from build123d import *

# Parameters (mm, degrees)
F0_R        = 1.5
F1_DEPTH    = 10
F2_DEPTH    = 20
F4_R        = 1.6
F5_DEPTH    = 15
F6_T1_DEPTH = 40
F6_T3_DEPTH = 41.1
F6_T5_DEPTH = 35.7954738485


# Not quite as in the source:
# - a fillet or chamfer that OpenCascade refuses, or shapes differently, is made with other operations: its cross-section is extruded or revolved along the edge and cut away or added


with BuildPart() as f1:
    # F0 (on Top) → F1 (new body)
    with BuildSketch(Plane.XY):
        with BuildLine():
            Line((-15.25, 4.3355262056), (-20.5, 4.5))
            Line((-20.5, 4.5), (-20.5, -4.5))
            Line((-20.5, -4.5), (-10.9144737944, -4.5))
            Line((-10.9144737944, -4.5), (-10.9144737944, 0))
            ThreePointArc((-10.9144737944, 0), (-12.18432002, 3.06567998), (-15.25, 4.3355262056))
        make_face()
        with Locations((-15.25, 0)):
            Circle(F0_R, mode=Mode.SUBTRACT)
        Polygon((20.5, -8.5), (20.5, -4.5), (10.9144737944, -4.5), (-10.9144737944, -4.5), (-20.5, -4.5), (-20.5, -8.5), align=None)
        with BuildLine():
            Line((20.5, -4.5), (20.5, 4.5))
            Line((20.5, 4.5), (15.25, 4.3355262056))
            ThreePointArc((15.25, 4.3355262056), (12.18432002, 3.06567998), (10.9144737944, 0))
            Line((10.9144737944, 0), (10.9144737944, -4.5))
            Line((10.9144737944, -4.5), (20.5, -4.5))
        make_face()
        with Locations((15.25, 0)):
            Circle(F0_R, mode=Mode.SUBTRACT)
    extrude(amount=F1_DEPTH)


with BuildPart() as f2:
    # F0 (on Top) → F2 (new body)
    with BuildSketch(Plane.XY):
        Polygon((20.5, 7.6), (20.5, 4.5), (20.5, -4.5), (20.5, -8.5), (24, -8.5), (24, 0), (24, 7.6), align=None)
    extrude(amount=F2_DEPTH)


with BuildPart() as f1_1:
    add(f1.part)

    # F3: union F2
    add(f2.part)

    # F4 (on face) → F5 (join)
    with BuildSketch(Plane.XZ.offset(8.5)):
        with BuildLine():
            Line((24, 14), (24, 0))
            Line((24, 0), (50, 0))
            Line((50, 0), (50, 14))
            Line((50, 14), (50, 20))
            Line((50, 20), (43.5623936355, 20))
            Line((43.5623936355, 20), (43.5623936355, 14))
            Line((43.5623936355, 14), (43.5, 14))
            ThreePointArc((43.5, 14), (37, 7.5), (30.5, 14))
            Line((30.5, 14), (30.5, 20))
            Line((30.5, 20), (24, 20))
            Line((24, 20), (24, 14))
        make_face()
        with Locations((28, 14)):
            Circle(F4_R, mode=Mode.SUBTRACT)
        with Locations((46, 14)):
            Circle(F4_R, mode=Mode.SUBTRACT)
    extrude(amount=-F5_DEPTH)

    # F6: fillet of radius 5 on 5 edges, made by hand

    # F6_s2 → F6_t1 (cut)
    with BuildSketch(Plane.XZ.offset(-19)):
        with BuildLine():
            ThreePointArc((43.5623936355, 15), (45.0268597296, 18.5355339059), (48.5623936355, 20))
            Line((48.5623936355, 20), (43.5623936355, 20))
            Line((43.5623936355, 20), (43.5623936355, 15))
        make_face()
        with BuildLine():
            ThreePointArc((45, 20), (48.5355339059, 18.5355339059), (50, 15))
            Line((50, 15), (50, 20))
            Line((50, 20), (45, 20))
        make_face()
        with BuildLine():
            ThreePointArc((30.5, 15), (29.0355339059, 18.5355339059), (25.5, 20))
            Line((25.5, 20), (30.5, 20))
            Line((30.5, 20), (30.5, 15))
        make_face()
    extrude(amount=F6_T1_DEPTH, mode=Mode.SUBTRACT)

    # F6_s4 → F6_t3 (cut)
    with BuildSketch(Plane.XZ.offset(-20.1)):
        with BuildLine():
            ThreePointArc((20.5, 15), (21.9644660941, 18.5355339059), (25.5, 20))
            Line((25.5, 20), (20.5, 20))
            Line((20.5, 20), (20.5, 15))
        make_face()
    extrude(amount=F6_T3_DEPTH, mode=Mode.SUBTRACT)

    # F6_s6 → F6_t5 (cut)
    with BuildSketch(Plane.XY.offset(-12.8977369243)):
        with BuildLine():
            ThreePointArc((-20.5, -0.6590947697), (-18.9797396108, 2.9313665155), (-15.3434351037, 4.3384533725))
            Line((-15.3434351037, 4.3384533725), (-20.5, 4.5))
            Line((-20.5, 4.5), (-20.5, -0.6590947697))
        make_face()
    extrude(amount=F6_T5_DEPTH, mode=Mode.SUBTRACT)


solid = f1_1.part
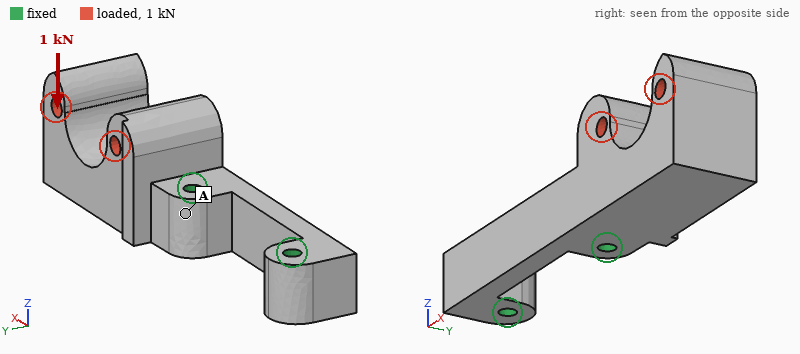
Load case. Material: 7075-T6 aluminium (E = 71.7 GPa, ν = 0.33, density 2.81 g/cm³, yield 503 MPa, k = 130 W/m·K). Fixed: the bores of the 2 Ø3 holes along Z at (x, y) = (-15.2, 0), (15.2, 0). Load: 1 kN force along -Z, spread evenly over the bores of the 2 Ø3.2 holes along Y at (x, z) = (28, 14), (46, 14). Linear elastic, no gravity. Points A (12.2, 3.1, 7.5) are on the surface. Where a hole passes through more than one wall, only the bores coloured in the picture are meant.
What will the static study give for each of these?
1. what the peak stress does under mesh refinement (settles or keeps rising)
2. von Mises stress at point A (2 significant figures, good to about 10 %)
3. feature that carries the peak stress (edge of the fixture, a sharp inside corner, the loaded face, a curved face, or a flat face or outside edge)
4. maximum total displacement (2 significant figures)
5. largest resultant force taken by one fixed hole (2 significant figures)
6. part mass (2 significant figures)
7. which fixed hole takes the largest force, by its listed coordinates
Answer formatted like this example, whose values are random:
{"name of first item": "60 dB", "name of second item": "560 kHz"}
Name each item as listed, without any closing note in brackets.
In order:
{"what the peak stress does under mesh refinement": "keeps rising", "von Mises stress at point A": "20 MPa", "feature that carries the peak stress": "edge of the fixture", "maximum total displacement": "0.11 mm", "largest resultant force taken by one fixed hole": "1.1 kN", "part mass": "26 g", "which fixed hole takes the largest force, by its listed coordinates": "(15.2, 0)"}
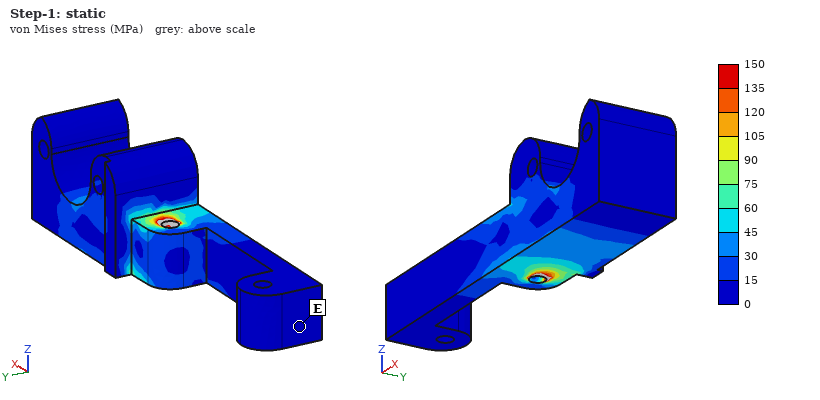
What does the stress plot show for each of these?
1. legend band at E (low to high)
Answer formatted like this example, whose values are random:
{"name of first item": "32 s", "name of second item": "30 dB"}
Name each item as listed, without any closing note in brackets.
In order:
{"legend band at E": "0 to 15 MPa"}
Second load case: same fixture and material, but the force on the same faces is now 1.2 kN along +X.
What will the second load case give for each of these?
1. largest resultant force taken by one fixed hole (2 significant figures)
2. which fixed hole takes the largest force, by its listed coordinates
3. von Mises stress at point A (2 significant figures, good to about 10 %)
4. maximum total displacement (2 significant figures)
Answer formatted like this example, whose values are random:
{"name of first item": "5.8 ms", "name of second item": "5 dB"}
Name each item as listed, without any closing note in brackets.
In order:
{"largest resultant force taken by one fixed hole": "1.1 kN", "which fixed hole takes the largest force, by its listed coordinates": "(15.2, 0)", "von Mises stress at point A": "14 MPa", "maximum total displacement": "84 µm"}
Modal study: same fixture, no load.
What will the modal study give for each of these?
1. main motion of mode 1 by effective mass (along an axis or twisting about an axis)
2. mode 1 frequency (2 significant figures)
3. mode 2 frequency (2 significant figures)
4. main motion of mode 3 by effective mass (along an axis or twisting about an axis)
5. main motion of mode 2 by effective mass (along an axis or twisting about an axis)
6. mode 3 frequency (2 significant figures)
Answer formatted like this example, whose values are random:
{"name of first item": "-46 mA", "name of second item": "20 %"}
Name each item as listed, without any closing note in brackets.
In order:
{"main motion of mode 1 by effective mass": "along Y", "mode 1 frequency": "4500 Hz", "mode 2 frequency": "4800 Hz", "main motion of mode 3 by effective mass": "twisting about X", "main motion of mode 2 by effective mass": "along Z", "mode 3 frequency": "12 kHz"}
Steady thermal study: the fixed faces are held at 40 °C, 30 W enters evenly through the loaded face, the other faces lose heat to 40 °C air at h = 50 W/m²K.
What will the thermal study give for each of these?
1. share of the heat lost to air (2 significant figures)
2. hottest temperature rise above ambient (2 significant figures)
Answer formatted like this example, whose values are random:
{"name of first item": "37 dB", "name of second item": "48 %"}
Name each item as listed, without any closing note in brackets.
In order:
{"share of the heat lost to air": "10 %", "hottest temperature rise above ambient": "40 K"}
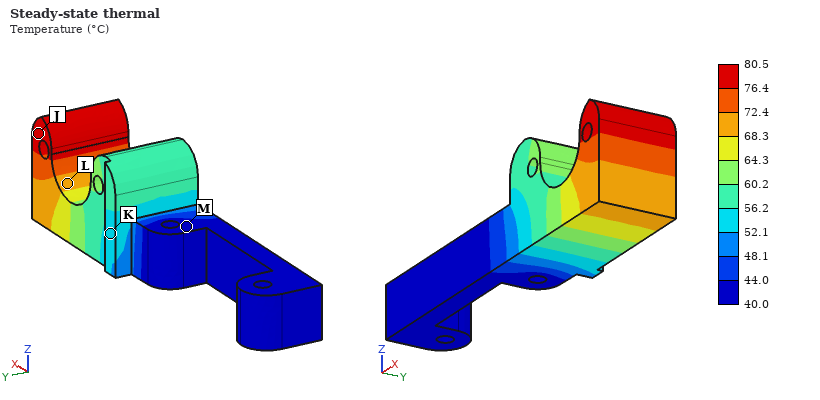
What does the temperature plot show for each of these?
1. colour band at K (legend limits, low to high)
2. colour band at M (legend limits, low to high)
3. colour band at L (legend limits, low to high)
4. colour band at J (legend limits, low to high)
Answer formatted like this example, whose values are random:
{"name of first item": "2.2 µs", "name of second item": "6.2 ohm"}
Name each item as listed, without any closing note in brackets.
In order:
{"colour band at K": "52.1 to 56.2 °C", "colour band at M": "40.0 to 44.0 °C", "colour band at L": "68.3 to 72.4 °C", "colour band at J": "76.4 to 80.5 °C"}
